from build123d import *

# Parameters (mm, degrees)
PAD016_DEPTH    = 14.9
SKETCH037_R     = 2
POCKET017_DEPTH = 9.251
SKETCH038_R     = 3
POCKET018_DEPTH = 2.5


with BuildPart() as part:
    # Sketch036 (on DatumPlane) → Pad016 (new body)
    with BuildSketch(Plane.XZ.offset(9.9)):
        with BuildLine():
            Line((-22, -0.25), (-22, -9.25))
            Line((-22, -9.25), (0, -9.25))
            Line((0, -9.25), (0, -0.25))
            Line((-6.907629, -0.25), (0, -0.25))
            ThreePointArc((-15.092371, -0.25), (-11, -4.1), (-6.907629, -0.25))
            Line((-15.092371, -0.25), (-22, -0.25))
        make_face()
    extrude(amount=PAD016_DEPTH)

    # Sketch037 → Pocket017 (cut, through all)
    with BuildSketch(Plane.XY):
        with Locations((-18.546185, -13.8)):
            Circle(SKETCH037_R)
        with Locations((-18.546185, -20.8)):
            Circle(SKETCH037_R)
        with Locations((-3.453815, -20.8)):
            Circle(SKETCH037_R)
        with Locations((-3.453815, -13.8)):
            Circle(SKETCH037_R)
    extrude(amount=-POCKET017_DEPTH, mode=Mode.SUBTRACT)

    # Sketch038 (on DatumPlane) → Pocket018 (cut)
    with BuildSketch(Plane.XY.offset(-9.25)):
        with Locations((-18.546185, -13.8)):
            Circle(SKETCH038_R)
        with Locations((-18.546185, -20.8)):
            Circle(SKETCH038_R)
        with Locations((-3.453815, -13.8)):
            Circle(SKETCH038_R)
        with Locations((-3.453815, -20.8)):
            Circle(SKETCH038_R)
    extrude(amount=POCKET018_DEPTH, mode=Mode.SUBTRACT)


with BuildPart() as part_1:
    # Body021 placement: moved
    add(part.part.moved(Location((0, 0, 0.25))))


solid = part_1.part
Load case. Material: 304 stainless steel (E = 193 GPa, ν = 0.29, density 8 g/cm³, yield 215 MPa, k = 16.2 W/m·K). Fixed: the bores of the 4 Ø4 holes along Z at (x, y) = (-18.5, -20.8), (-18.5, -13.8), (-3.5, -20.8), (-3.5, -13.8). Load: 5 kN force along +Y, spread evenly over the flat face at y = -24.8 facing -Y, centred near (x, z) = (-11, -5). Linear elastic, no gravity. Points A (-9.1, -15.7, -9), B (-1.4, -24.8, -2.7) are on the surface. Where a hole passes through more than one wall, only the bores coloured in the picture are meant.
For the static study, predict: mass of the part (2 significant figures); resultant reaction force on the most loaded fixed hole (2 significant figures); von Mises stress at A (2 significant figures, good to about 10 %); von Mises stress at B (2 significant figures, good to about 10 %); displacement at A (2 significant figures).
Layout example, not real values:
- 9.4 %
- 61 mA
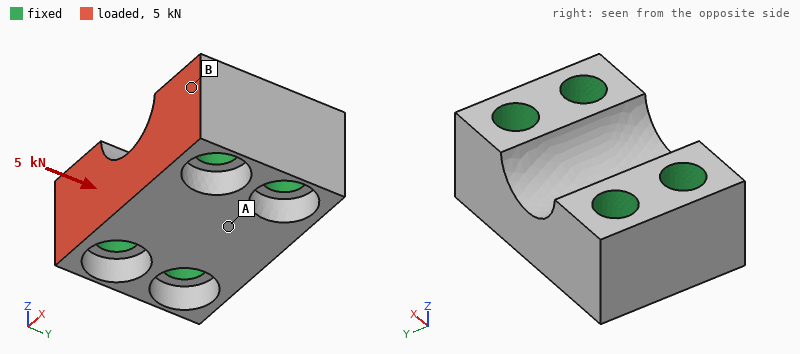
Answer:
- 16 g
- 2.0 kN
- 16 MPa
- 36 MPa
- 0.87 µm
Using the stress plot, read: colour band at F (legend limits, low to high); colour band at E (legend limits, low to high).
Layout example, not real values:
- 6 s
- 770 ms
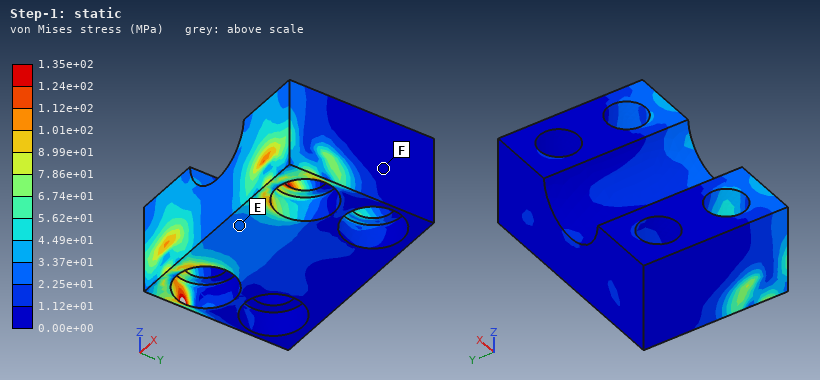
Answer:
- 0.00e+00 to 1.12e+01 MPa
- 2.25e+01 to 3.37e+01 MPa
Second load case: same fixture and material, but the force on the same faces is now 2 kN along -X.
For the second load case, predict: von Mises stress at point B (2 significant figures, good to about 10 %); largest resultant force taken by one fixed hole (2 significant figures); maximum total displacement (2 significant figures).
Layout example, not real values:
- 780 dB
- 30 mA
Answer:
- 26 MPa
- 1.0 kN
- 1.7 µm
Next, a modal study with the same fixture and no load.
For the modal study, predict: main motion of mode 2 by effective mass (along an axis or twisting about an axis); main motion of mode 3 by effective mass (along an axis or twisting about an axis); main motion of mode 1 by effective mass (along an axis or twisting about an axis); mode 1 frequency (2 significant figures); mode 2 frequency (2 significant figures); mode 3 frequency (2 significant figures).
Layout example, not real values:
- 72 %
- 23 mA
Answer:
- along Z
- along Y
- along Y
- 86 kHz
- 100 kHz
- 120 kHz
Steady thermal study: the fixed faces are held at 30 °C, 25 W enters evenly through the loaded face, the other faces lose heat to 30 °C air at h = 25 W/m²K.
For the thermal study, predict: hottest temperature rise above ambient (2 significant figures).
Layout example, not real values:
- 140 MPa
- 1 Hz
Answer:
- 57 K
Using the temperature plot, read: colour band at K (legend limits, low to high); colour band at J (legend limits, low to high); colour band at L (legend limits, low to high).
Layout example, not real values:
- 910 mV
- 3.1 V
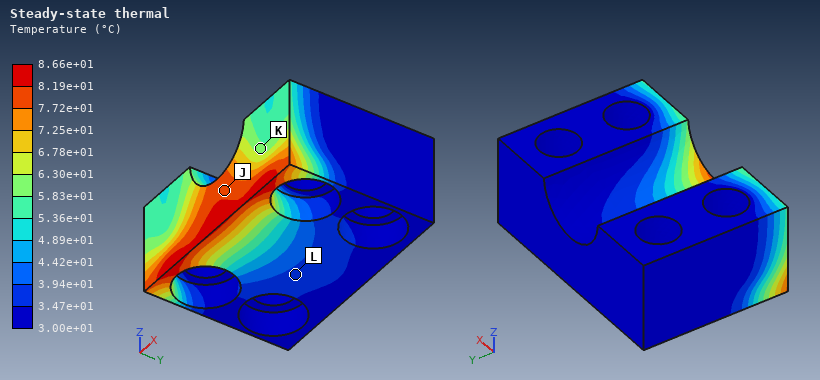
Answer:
- 5.83e+01 to 6.30e+01 °C
- 7.72e+01 to 8.19e+01 °C
- 3.47e+01 to 3.94e+01 °C
